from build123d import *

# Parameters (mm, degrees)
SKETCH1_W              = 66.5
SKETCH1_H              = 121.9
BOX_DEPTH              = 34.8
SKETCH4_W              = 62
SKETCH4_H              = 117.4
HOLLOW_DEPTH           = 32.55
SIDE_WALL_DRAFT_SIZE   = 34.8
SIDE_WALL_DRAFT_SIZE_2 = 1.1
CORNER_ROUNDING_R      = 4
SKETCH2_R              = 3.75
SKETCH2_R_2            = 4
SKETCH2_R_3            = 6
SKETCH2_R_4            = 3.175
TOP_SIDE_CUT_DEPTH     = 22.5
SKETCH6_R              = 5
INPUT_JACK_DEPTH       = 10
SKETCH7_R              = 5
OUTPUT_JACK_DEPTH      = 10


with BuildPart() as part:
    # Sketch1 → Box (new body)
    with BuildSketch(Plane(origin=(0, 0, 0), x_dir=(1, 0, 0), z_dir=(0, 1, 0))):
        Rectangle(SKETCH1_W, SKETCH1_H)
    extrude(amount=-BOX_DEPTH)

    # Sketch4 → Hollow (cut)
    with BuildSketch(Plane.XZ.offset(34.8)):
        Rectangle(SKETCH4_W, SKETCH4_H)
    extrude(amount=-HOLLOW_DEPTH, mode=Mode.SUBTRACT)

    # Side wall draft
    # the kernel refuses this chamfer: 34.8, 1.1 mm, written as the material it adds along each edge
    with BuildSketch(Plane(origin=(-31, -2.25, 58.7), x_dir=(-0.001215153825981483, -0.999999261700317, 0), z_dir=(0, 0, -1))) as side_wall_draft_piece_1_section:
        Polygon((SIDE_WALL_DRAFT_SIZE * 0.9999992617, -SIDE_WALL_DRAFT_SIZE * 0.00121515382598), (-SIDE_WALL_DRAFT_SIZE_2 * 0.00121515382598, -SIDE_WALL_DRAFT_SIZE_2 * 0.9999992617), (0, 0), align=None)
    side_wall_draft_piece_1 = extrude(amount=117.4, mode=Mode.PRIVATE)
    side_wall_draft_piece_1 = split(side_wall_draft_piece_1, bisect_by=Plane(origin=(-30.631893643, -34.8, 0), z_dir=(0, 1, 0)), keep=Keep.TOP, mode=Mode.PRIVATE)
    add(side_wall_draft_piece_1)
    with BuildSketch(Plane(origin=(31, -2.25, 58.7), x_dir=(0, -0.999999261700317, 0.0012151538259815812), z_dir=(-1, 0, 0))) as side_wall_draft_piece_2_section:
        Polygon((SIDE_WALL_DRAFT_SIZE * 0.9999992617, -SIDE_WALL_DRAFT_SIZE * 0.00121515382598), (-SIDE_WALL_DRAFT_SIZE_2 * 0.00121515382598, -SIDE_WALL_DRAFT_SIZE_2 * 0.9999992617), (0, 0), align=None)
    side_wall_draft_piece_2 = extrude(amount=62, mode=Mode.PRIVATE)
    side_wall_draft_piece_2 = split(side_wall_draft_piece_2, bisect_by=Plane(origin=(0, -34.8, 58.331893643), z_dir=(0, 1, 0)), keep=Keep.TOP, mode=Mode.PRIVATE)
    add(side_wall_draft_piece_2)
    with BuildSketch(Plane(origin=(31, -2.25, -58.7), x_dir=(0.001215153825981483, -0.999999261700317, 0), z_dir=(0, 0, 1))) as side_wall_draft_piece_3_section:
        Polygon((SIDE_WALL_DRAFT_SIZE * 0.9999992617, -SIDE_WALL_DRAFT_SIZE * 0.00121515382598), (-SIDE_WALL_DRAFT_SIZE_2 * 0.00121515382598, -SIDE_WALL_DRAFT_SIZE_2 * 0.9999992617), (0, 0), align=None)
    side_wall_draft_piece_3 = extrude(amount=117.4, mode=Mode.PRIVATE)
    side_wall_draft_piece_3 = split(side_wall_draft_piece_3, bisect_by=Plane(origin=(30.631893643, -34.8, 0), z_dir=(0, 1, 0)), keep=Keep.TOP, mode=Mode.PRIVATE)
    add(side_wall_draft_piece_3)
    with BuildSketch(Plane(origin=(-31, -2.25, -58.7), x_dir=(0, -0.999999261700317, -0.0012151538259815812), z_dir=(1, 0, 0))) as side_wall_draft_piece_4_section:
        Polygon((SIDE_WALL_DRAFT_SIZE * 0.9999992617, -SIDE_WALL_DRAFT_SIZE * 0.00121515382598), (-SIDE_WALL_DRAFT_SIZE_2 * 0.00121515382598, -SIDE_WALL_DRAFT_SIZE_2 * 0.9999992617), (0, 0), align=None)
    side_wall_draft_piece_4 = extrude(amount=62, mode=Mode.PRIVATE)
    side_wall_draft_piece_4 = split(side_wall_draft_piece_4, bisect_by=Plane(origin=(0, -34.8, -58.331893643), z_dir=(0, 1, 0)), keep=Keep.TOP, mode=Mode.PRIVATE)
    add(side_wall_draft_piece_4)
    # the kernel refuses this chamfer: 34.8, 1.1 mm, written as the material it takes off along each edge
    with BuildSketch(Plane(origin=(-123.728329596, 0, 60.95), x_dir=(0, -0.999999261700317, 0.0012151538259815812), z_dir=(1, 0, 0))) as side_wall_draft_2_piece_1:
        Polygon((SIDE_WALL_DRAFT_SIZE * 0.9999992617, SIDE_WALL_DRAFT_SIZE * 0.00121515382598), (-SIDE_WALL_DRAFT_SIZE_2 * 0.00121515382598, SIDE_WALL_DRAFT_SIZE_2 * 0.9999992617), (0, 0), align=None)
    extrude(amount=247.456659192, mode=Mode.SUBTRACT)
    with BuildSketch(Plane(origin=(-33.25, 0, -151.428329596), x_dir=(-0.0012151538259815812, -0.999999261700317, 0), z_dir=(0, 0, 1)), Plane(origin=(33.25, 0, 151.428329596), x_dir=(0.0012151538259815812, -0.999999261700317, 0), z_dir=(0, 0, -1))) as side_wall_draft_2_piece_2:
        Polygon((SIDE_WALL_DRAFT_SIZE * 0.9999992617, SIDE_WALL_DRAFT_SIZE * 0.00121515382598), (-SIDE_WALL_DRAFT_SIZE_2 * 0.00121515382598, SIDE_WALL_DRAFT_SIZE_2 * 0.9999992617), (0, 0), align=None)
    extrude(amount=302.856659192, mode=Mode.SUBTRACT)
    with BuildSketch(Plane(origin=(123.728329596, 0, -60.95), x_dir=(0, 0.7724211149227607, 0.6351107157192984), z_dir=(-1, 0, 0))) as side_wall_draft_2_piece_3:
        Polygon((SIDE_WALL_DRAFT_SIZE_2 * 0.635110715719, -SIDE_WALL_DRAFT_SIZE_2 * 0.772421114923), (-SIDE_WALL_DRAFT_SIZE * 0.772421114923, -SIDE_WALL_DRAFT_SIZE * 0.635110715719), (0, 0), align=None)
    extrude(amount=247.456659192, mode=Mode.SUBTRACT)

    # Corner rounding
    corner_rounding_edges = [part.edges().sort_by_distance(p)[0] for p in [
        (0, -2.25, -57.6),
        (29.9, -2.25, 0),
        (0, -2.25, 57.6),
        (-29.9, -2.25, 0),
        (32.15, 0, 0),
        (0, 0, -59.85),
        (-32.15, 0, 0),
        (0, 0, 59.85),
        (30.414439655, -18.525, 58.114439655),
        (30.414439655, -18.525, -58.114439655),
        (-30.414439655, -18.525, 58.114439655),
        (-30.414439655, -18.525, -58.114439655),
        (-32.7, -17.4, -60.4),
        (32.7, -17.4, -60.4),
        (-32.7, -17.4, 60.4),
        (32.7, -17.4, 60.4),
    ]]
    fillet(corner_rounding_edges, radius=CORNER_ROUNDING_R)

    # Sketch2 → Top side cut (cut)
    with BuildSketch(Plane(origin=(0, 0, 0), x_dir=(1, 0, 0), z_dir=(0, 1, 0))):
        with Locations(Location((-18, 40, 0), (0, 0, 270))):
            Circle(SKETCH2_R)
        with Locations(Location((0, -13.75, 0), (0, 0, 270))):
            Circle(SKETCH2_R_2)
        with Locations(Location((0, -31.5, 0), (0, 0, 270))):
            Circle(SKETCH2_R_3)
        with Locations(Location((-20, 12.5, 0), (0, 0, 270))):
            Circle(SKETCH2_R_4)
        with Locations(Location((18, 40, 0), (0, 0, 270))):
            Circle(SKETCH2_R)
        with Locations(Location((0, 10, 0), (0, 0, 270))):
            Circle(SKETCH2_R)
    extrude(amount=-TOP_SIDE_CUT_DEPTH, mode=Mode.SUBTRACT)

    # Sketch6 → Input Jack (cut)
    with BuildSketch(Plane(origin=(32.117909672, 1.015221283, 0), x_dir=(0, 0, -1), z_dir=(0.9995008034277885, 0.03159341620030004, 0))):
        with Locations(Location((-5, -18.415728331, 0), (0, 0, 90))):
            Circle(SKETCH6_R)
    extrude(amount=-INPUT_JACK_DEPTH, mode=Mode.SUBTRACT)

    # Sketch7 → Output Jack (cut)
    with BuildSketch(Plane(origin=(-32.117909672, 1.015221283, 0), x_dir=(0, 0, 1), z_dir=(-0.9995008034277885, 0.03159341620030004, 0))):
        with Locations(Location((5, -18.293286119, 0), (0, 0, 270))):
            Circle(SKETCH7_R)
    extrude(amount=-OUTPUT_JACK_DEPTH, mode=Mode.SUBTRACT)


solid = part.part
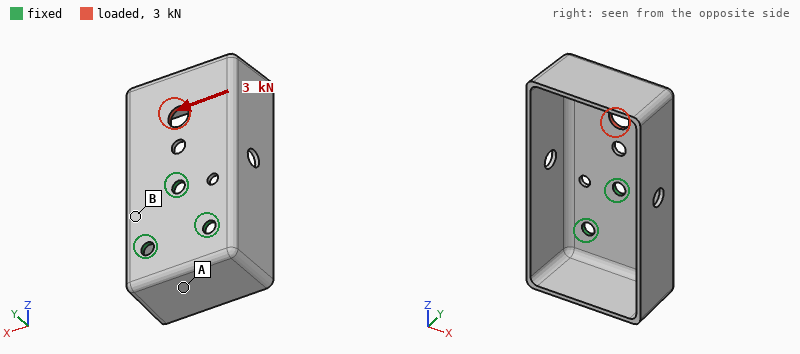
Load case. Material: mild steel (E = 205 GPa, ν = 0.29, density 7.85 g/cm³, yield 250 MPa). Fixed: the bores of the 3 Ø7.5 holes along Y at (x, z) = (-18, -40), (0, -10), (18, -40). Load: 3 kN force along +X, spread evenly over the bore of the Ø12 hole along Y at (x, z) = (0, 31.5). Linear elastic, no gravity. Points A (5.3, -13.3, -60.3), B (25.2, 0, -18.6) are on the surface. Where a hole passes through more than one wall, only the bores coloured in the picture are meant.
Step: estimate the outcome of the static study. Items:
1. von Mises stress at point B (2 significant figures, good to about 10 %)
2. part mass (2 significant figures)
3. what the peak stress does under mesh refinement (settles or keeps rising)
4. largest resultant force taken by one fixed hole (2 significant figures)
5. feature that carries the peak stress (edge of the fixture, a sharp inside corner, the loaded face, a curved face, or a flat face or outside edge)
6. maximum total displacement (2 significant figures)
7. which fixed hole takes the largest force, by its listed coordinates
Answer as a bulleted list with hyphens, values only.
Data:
- 41 MPa
- 340 g
- keeps rising
- 4.1 kN
- edge of the fixture
- 63 µm
- (0, -10)
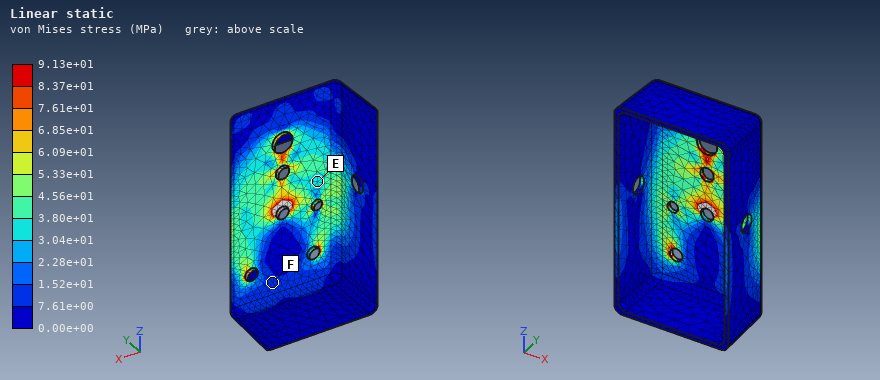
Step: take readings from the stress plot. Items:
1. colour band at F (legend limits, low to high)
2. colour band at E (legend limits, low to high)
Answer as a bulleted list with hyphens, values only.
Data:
- 7.61e+00 to 1.52e+01 MPa
- 3.04e+01 to 3.80e+01 MPa
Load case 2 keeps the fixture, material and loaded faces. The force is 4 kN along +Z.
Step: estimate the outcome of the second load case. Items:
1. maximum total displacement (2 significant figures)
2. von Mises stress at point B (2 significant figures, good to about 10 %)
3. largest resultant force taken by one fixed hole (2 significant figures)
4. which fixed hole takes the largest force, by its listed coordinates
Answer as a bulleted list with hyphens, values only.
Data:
- 13 µm
- 17 MPa
- 2.2 kN
- (0, -10)
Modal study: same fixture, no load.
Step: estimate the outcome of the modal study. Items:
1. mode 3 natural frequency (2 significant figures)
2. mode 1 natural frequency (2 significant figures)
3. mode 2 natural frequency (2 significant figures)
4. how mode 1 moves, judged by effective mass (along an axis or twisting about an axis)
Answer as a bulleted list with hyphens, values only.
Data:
- 1800 Hz
- 470 Hz
- 550 Hz
- along Y
